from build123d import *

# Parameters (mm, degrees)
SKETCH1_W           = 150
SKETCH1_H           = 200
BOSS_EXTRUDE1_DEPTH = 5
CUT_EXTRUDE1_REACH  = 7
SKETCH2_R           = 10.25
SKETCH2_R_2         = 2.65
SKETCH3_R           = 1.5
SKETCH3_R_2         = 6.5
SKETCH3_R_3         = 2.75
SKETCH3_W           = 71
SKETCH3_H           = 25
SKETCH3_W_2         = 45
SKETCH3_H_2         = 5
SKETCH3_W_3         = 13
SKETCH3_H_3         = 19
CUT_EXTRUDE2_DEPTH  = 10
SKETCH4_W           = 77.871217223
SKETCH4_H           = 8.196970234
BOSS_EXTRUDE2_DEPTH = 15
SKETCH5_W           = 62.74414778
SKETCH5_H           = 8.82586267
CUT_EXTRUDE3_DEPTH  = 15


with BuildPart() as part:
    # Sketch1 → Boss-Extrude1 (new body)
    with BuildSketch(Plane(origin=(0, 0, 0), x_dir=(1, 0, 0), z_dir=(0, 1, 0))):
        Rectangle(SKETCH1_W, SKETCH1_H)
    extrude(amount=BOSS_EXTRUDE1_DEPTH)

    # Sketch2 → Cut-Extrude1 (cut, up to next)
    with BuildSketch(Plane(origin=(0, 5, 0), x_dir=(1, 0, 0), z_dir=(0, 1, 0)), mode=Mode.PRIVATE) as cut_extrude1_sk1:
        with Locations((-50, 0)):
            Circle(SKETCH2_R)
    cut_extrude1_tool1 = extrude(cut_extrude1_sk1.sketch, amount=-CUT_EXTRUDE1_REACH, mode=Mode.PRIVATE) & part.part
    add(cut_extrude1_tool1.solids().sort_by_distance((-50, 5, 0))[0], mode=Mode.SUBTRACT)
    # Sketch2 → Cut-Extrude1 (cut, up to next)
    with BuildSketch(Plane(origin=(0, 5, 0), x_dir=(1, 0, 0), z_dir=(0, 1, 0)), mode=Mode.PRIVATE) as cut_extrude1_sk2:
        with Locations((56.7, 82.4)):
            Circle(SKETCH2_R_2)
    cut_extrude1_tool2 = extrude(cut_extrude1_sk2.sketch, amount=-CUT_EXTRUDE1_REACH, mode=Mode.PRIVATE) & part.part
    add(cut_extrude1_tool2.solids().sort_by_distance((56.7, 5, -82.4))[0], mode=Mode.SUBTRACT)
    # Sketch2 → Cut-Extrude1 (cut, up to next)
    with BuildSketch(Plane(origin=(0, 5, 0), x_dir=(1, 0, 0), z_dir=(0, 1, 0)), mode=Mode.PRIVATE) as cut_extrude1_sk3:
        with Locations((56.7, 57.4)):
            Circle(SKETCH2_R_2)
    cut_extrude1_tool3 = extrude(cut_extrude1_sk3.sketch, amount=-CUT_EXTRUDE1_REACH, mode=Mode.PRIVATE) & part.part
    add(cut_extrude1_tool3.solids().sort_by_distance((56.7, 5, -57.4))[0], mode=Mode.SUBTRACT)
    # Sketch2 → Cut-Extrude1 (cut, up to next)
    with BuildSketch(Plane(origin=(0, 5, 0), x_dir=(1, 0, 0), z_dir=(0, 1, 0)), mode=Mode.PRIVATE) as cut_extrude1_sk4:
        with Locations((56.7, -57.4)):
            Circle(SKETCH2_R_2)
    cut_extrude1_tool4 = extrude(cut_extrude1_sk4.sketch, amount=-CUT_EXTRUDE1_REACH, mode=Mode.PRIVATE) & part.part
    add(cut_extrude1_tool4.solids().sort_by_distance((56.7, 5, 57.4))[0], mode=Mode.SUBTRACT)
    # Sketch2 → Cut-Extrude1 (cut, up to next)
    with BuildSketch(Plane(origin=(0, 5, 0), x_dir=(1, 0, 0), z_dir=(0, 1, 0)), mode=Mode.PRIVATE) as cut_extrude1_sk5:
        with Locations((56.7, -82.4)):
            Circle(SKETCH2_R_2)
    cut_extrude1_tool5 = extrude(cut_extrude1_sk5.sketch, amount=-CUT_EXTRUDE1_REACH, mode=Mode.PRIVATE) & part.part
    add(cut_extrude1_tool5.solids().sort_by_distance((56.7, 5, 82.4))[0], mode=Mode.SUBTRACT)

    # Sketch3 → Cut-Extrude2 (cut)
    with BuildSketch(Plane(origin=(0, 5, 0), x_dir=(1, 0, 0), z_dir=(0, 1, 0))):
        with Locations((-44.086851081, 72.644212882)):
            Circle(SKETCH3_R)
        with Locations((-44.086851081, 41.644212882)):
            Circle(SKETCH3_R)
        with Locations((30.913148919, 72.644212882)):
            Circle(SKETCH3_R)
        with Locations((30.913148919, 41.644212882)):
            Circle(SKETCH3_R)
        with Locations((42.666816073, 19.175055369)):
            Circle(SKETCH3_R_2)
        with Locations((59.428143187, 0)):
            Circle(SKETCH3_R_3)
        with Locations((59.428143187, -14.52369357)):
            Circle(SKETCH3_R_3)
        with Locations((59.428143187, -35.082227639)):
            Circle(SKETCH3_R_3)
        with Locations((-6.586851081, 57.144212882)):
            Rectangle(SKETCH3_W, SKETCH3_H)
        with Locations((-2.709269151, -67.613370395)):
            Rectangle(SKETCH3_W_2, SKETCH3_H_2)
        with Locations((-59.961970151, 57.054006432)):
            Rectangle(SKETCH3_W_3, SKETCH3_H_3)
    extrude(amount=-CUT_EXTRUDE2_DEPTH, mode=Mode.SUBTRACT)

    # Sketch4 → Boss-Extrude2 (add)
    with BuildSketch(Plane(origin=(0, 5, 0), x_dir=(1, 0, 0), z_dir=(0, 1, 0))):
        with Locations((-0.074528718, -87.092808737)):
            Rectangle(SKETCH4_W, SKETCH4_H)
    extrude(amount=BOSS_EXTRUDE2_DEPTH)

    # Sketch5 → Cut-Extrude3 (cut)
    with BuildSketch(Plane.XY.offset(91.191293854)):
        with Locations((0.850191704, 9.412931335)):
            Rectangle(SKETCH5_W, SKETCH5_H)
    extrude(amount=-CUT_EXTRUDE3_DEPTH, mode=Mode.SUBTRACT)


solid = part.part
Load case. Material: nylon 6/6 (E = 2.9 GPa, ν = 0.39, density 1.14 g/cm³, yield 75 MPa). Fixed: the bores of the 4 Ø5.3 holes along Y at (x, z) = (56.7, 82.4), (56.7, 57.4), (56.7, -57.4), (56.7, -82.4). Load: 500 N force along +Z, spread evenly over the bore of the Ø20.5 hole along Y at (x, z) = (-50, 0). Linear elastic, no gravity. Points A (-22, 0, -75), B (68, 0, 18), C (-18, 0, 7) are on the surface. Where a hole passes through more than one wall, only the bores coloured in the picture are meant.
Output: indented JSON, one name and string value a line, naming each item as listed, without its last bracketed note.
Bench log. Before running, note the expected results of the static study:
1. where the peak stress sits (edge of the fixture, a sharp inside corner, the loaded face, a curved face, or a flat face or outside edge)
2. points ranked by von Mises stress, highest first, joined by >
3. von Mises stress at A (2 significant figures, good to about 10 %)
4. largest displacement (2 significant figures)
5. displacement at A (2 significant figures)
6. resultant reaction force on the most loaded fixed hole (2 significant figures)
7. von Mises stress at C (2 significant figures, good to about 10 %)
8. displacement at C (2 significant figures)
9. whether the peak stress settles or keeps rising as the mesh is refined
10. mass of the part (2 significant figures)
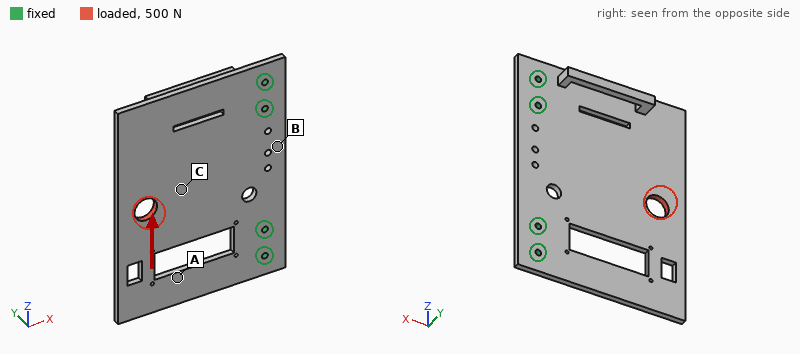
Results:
{
  "where the peak stress sits": "a sharp inside corner",
  "points ranked by von Mises stress, highest first, joined by >": "C > A > B",
  "von Mises stress at A": "0.89 MPa",
  "largest displacement": "0.18 mm",
  "displacement at A": "0.11 mm",
  "resultant reaction force on the most loaded fixed hole": "320 N",
  "von Mises stress at C": "1.8 MPa",
  "displacement at C": "0.099 mm",
  "whether the peak stress settles or keeps rising as the mesh is refined": "keeps rising",
  "mass of the part": "160 g"
}
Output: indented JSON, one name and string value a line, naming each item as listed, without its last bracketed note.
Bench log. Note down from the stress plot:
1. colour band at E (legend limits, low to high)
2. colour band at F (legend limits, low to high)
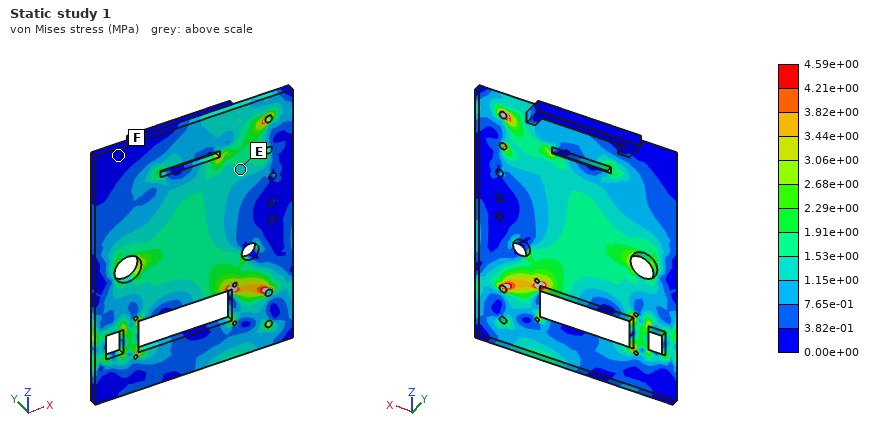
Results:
{
  "colour band at E": "1.15e+00 to 1.53e+00 MPa",
  "colour band at F": "0.00e+00 to 3.82e-01 MPa"
}
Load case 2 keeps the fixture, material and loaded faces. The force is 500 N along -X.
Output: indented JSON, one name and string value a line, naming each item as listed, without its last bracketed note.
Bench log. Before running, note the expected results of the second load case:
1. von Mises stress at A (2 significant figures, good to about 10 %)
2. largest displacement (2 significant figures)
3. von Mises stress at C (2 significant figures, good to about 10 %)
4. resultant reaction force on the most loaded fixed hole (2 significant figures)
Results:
{
  "von Mises stress at A": "0.56 MPa",
  "largest displacement": "89 µm",
  "von Mises stress at C": "1.3 MPa",
  "resultant reaction force on the most loaded fixed hole": "230 N"
}
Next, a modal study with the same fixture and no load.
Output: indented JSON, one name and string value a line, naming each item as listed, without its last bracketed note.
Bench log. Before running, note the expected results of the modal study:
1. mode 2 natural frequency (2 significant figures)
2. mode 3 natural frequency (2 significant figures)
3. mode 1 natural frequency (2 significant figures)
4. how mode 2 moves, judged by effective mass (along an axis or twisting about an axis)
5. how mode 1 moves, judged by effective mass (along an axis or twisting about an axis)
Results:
{
  "mode 2 natural frequency": "130 Hz",
  "mode 3 natural frequency": "260 Hz",
  "mode 1 natural frequency": "72 Hz",
  "how mode 2 moves, judged by effective mass": "twisting about X",
  "how mode 1 moves, judged by effective mass": "along Y"
}
